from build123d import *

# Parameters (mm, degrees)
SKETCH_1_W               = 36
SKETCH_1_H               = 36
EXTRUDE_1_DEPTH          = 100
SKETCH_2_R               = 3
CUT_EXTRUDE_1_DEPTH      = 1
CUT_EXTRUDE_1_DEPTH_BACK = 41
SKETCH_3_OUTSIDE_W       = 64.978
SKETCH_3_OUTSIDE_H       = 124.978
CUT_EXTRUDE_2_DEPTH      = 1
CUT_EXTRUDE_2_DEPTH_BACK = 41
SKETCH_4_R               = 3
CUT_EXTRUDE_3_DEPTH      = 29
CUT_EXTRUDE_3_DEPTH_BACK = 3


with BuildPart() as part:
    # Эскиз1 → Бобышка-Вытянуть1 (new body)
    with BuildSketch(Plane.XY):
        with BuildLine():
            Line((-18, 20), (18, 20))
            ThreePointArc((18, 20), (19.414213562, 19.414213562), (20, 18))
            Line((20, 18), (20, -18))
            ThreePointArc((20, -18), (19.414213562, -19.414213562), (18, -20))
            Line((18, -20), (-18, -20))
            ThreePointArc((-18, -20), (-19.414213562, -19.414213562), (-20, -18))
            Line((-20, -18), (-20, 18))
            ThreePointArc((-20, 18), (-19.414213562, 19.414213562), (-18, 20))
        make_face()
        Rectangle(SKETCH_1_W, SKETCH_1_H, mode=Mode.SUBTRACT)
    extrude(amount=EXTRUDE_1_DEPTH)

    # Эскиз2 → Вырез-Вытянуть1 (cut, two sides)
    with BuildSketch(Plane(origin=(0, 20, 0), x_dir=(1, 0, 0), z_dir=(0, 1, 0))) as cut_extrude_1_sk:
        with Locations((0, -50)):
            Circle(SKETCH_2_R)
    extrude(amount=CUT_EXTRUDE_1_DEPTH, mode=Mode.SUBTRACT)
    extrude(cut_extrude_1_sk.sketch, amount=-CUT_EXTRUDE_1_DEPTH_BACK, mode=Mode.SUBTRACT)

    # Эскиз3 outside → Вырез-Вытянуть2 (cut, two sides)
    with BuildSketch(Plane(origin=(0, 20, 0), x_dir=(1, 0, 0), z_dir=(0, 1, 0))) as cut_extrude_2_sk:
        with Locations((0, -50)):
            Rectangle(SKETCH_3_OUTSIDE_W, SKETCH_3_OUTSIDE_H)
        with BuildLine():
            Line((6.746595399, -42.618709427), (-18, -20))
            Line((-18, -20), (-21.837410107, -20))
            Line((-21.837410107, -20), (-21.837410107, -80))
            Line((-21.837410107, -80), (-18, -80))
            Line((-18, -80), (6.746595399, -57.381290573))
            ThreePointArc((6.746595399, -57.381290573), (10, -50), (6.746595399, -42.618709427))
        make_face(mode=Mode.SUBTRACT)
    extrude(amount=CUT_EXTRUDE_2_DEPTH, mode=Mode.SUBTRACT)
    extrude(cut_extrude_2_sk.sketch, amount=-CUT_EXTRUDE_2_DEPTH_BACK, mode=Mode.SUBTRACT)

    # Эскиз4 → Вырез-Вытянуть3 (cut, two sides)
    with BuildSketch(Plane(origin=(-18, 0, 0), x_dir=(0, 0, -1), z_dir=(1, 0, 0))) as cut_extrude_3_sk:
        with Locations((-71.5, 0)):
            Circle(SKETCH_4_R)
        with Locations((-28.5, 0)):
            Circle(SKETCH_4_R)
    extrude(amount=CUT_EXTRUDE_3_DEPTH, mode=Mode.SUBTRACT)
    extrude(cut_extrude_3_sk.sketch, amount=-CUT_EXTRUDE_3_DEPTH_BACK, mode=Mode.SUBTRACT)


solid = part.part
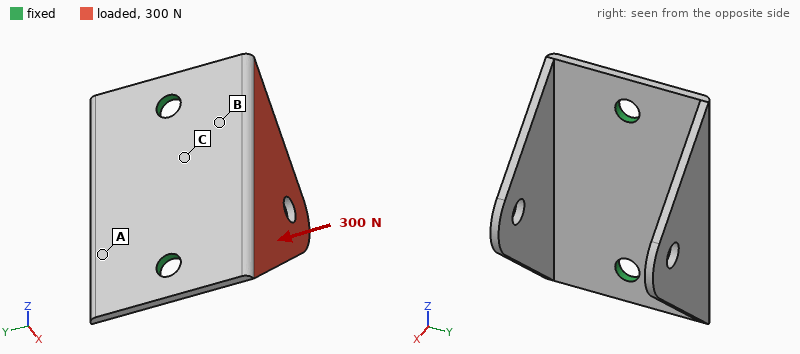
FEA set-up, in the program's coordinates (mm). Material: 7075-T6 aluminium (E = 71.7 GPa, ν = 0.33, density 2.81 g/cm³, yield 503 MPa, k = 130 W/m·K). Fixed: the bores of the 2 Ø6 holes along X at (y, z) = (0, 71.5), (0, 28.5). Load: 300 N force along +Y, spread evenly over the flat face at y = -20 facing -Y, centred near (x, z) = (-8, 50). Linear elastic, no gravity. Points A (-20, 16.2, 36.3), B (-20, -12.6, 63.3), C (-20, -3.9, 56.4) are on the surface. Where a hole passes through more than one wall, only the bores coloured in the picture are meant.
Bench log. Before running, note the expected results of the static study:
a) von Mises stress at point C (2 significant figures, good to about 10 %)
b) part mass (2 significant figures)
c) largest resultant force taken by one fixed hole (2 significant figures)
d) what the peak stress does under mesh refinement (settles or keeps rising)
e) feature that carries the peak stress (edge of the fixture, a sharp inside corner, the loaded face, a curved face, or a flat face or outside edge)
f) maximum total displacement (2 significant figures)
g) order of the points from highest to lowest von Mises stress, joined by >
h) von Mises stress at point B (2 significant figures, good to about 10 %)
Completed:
47 MPa
23 g
150 N
keeps rising
edge of the fixture
0.88 mm
B > C > A
75 MPa
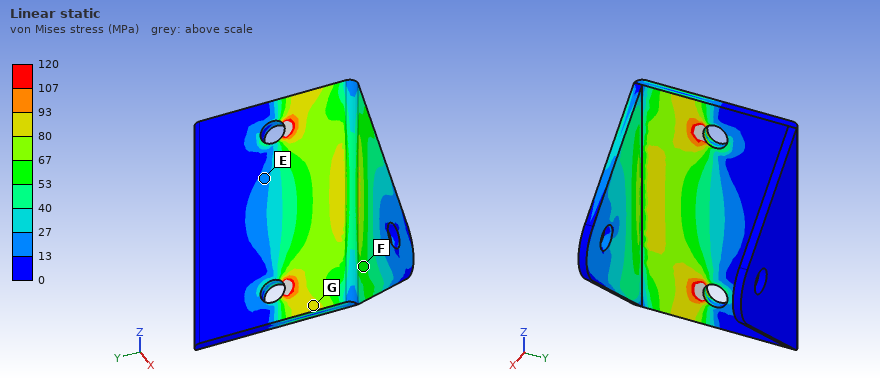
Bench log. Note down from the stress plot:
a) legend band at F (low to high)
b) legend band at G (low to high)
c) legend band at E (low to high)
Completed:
53 to 67 MPa
80 to 93 MPa
13 to 27 MPa
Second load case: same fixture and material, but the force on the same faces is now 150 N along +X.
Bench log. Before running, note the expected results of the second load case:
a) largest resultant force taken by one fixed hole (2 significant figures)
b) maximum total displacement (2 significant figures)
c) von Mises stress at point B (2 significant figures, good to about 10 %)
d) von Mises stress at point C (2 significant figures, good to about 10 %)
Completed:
75 N
0.30 mm
27 MPa
28 MPa
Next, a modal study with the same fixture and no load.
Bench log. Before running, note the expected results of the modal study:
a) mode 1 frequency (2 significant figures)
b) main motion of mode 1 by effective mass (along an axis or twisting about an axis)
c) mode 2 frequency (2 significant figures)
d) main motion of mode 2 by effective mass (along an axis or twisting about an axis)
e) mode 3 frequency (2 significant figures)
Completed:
1500 Hz
along Y
1600 Hz
along X
3200 Hz
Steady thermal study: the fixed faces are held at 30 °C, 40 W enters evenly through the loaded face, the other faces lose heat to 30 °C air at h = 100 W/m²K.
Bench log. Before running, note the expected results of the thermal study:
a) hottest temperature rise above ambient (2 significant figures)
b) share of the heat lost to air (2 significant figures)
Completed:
79 K
36 %
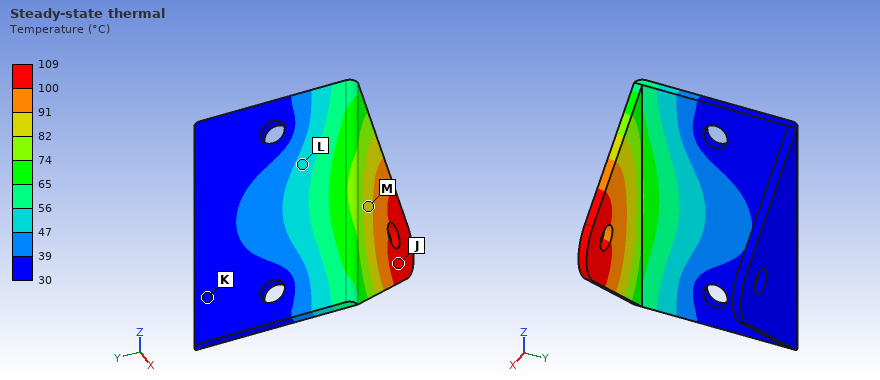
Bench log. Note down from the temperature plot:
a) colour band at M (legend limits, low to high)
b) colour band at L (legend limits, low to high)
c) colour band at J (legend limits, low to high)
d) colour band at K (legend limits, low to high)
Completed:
82 to 91 °C
47 to 56 °C
100 to 109 °C
30 to 39 °C
